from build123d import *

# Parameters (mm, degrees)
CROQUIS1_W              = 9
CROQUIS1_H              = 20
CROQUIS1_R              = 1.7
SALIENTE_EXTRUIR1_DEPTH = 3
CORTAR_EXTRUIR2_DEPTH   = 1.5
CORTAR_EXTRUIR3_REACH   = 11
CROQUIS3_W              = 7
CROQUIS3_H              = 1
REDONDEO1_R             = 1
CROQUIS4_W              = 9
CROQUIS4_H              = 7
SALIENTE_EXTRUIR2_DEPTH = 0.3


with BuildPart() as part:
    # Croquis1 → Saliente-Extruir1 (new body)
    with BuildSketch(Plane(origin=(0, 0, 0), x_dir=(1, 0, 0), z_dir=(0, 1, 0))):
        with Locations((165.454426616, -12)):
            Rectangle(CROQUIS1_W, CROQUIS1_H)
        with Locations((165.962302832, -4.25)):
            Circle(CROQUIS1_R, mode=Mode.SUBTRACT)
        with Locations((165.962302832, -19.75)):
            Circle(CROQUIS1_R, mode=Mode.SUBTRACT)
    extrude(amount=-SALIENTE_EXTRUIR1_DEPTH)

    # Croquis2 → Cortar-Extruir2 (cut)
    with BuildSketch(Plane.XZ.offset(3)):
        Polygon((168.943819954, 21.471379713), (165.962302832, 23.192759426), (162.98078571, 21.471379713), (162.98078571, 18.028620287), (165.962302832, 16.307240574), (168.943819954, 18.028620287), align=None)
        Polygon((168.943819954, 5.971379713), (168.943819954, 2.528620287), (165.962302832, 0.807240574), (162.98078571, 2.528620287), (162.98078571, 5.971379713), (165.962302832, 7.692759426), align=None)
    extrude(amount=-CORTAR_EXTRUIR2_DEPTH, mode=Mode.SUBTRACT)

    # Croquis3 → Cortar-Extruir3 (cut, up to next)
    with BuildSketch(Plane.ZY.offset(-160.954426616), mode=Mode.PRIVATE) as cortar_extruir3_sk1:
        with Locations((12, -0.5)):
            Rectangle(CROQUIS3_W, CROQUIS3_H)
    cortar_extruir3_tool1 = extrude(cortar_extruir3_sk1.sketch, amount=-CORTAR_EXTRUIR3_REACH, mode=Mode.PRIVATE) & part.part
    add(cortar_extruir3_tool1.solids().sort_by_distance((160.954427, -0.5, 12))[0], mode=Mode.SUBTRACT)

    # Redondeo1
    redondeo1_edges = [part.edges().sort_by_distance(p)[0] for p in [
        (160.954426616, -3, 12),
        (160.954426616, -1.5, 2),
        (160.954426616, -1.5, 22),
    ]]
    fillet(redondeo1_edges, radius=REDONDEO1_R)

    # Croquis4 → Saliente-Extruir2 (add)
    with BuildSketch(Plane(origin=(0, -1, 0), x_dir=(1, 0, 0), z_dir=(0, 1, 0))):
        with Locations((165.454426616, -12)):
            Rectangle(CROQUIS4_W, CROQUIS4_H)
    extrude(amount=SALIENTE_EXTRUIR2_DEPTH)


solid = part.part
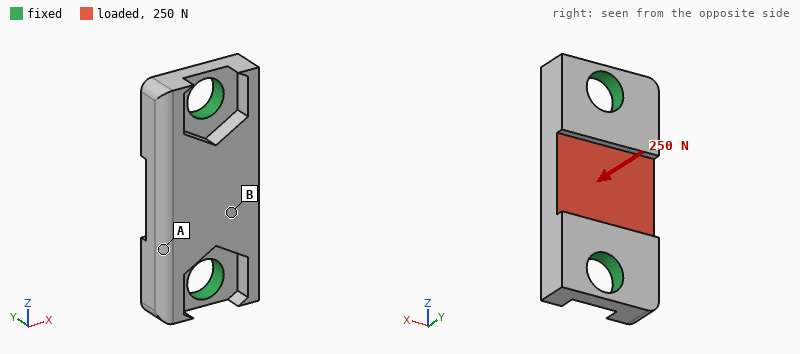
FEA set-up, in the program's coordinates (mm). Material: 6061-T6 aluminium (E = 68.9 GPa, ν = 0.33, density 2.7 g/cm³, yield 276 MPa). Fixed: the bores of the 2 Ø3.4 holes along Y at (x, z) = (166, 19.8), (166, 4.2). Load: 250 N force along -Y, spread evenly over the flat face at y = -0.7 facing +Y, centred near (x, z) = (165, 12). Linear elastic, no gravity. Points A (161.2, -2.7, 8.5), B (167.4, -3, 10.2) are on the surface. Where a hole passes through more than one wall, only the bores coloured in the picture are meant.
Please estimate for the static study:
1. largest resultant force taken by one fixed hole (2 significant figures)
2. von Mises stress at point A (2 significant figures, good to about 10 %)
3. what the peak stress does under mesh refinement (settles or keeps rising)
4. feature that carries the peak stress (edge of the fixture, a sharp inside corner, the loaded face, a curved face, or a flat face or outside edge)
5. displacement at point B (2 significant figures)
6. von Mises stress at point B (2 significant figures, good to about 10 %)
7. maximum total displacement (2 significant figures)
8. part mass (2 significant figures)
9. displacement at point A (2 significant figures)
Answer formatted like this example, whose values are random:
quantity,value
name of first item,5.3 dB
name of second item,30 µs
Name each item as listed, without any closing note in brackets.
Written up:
quantity,value
largest resultant force taken by one fixed hole,190 N
von Mises stress at point A,12 MPa
what the peak stress does under mesh refinement,keeps rising
feature that carries the peak stress,edge of the fixture
displacement at point B,4.9 µm
von Mises stress at point B,29 MPa
maximum total displacement,8.7 µm
part mass,1.0 g
displacement at point A,6.1 µm
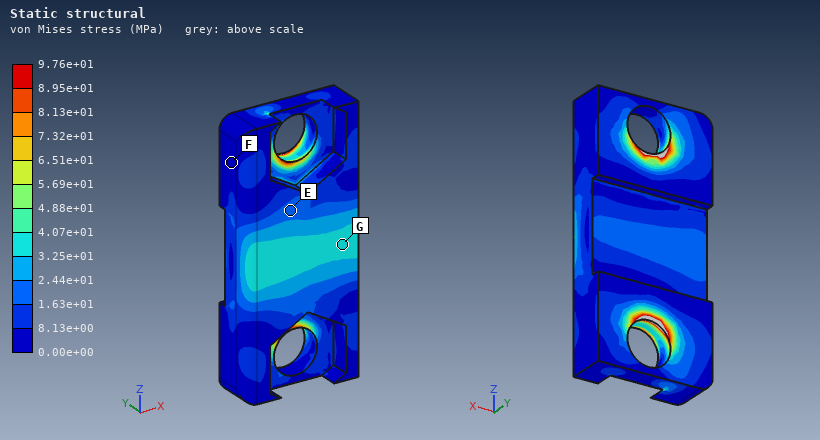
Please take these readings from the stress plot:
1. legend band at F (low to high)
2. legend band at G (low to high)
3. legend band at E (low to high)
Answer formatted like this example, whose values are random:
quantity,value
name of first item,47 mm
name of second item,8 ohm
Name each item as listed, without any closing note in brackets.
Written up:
quantity,value
legend band at F,0.00e+00 to 8.13e+00 MPa
legend band at G,3.25e+01 to 4.07e+01 MPa
legend band at E,1.63e+01 to 2.44e+01 MPa
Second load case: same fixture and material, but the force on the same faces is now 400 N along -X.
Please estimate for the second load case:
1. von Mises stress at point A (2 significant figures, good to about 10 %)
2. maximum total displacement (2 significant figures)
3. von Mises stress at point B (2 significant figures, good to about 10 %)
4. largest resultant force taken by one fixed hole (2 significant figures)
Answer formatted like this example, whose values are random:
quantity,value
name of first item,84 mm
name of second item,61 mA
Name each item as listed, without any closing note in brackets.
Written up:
quantity,value
von Mises stress at point A,11 MPa
maximum total displacement,4.8 µm
von Mises stress at point B,9.0 MPa
largest resultant force taken by one fixed hole,200 N
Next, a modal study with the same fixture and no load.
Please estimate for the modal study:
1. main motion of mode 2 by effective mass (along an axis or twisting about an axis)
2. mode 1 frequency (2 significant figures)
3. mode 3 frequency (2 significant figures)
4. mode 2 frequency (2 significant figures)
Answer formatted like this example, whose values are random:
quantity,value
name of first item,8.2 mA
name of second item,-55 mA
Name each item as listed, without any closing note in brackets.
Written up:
quantity,value
main motion of mode 2 by effective mass,along Y
mode 1 frequency,38 kHz
mode 3 frequency,70 kHz
mode 2 frequency,50 kHz
